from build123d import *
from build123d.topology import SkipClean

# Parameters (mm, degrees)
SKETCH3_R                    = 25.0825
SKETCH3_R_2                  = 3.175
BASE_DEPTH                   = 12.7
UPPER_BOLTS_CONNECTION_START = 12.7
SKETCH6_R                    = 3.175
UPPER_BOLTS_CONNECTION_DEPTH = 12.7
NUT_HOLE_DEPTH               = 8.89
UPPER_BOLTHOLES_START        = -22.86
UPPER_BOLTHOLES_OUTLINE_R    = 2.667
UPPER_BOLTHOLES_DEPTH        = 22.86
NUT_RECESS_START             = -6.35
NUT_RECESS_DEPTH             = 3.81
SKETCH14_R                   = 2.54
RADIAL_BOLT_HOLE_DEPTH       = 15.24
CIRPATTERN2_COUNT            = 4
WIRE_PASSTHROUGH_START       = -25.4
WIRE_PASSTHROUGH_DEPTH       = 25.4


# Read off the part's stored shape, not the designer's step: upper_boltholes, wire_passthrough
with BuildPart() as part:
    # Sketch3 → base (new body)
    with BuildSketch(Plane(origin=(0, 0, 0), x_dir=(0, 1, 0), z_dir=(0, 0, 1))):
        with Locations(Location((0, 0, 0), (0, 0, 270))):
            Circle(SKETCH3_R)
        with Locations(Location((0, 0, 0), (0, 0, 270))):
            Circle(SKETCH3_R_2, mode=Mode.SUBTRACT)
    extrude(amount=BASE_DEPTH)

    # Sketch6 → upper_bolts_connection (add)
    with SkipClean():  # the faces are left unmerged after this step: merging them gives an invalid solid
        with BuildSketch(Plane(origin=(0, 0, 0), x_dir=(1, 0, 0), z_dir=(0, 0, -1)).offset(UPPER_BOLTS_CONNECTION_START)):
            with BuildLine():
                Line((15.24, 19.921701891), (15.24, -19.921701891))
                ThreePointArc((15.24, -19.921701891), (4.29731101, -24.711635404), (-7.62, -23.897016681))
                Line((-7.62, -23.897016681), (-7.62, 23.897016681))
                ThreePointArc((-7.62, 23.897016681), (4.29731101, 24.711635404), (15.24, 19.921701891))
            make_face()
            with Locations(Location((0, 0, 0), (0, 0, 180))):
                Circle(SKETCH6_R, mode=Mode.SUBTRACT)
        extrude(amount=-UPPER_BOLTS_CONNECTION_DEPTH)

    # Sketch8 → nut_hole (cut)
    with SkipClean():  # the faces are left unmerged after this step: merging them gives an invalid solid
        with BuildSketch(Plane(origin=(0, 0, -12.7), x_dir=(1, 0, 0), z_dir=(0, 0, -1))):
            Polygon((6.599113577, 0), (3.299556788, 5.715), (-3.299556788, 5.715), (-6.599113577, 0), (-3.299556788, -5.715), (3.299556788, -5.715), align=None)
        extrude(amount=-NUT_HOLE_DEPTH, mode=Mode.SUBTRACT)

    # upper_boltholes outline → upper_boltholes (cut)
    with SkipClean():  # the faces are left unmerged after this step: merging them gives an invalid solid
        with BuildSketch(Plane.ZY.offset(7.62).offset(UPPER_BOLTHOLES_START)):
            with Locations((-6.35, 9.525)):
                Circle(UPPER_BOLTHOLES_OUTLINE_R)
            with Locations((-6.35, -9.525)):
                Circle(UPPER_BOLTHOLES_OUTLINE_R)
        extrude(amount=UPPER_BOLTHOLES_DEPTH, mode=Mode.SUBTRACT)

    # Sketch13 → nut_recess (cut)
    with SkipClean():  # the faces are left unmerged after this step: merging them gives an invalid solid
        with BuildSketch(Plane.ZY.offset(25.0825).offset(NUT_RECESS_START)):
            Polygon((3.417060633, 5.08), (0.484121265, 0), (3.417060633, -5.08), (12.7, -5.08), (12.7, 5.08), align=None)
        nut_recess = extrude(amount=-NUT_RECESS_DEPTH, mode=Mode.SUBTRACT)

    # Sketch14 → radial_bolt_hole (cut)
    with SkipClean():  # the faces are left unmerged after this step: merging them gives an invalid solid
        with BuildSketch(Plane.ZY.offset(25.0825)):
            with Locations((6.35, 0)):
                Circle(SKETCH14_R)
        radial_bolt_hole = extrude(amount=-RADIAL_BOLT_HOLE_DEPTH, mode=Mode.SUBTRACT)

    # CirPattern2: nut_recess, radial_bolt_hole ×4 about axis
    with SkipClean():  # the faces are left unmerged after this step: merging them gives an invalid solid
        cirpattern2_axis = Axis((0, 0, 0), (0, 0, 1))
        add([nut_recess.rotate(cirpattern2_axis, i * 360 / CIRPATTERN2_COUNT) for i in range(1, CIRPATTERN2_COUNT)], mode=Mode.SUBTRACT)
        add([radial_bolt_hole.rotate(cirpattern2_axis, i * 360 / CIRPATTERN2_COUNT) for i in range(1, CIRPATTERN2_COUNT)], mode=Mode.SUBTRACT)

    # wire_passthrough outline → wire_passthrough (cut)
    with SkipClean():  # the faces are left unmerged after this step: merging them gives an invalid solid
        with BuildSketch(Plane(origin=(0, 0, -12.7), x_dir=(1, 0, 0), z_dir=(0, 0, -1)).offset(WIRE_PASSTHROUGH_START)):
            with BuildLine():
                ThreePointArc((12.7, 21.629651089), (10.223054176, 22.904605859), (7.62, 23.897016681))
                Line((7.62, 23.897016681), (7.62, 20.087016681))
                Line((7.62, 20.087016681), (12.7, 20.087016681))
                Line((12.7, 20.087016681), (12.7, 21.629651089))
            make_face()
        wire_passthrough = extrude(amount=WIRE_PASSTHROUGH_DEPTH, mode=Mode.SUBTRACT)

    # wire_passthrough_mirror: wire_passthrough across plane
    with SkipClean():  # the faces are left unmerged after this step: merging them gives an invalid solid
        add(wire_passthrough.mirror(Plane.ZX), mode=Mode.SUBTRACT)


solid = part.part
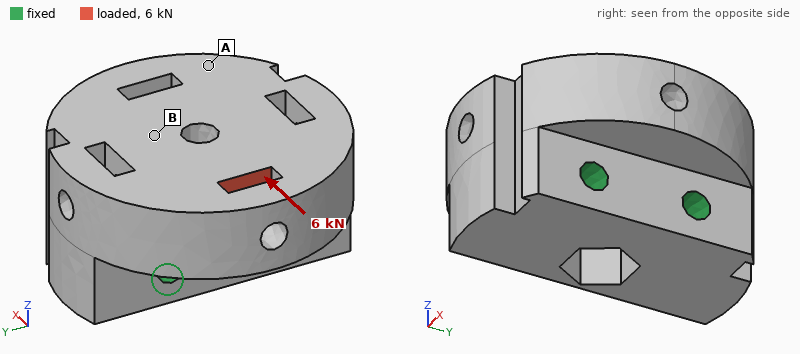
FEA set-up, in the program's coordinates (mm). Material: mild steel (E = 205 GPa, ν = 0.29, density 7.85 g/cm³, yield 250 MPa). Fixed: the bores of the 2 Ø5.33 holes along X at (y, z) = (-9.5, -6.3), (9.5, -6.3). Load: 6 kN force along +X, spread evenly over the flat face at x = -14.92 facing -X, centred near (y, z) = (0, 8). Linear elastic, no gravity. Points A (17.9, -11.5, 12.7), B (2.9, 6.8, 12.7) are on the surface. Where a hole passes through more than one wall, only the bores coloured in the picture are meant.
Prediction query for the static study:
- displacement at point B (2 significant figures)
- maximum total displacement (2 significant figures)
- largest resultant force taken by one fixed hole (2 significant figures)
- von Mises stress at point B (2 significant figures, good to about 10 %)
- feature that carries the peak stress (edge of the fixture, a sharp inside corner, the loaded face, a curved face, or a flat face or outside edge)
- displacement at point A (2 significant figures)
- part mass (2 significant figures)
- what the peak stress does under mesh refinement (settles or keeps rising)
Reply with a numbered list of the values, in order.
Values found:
1. 2.9 µm
2. 8.2 µm
3. 3.0 kN
4. 17 MPa
5. edge of the fixture
6. 2.9 µm
7. 260 g
8. keeps rising
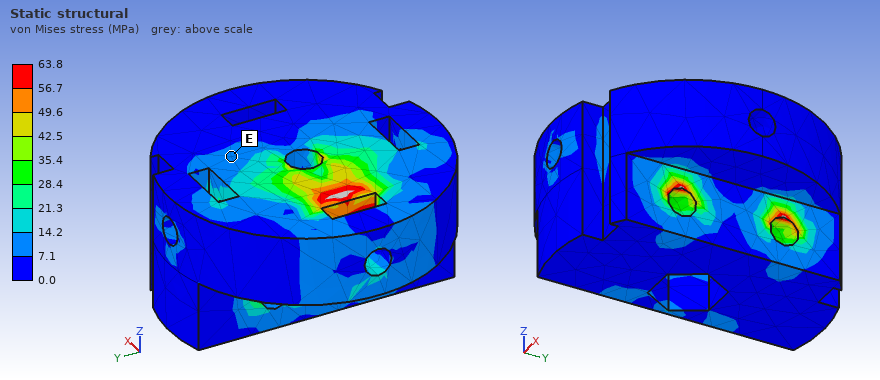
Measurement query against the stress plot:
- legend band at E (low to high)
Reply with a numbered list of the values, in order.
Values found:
1. 7.1 to 14.2 MPa
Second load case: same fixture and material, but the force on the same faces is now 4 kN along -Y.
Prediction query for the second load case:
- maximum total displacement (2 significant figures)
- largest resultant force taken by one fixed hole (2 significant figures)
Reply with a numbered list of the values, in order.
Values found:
1. 5.1 µm
2. 3.3 kN
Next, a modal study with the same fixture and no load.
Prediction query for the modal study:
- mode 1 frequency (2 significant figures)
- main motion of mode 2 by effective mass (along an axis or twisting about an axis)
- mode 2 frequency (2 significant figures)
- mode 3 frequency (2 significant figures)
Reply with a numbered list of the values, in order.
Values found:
1. 15 kHz
2. along Y
3. 18 kHz
4. 21 kHz
